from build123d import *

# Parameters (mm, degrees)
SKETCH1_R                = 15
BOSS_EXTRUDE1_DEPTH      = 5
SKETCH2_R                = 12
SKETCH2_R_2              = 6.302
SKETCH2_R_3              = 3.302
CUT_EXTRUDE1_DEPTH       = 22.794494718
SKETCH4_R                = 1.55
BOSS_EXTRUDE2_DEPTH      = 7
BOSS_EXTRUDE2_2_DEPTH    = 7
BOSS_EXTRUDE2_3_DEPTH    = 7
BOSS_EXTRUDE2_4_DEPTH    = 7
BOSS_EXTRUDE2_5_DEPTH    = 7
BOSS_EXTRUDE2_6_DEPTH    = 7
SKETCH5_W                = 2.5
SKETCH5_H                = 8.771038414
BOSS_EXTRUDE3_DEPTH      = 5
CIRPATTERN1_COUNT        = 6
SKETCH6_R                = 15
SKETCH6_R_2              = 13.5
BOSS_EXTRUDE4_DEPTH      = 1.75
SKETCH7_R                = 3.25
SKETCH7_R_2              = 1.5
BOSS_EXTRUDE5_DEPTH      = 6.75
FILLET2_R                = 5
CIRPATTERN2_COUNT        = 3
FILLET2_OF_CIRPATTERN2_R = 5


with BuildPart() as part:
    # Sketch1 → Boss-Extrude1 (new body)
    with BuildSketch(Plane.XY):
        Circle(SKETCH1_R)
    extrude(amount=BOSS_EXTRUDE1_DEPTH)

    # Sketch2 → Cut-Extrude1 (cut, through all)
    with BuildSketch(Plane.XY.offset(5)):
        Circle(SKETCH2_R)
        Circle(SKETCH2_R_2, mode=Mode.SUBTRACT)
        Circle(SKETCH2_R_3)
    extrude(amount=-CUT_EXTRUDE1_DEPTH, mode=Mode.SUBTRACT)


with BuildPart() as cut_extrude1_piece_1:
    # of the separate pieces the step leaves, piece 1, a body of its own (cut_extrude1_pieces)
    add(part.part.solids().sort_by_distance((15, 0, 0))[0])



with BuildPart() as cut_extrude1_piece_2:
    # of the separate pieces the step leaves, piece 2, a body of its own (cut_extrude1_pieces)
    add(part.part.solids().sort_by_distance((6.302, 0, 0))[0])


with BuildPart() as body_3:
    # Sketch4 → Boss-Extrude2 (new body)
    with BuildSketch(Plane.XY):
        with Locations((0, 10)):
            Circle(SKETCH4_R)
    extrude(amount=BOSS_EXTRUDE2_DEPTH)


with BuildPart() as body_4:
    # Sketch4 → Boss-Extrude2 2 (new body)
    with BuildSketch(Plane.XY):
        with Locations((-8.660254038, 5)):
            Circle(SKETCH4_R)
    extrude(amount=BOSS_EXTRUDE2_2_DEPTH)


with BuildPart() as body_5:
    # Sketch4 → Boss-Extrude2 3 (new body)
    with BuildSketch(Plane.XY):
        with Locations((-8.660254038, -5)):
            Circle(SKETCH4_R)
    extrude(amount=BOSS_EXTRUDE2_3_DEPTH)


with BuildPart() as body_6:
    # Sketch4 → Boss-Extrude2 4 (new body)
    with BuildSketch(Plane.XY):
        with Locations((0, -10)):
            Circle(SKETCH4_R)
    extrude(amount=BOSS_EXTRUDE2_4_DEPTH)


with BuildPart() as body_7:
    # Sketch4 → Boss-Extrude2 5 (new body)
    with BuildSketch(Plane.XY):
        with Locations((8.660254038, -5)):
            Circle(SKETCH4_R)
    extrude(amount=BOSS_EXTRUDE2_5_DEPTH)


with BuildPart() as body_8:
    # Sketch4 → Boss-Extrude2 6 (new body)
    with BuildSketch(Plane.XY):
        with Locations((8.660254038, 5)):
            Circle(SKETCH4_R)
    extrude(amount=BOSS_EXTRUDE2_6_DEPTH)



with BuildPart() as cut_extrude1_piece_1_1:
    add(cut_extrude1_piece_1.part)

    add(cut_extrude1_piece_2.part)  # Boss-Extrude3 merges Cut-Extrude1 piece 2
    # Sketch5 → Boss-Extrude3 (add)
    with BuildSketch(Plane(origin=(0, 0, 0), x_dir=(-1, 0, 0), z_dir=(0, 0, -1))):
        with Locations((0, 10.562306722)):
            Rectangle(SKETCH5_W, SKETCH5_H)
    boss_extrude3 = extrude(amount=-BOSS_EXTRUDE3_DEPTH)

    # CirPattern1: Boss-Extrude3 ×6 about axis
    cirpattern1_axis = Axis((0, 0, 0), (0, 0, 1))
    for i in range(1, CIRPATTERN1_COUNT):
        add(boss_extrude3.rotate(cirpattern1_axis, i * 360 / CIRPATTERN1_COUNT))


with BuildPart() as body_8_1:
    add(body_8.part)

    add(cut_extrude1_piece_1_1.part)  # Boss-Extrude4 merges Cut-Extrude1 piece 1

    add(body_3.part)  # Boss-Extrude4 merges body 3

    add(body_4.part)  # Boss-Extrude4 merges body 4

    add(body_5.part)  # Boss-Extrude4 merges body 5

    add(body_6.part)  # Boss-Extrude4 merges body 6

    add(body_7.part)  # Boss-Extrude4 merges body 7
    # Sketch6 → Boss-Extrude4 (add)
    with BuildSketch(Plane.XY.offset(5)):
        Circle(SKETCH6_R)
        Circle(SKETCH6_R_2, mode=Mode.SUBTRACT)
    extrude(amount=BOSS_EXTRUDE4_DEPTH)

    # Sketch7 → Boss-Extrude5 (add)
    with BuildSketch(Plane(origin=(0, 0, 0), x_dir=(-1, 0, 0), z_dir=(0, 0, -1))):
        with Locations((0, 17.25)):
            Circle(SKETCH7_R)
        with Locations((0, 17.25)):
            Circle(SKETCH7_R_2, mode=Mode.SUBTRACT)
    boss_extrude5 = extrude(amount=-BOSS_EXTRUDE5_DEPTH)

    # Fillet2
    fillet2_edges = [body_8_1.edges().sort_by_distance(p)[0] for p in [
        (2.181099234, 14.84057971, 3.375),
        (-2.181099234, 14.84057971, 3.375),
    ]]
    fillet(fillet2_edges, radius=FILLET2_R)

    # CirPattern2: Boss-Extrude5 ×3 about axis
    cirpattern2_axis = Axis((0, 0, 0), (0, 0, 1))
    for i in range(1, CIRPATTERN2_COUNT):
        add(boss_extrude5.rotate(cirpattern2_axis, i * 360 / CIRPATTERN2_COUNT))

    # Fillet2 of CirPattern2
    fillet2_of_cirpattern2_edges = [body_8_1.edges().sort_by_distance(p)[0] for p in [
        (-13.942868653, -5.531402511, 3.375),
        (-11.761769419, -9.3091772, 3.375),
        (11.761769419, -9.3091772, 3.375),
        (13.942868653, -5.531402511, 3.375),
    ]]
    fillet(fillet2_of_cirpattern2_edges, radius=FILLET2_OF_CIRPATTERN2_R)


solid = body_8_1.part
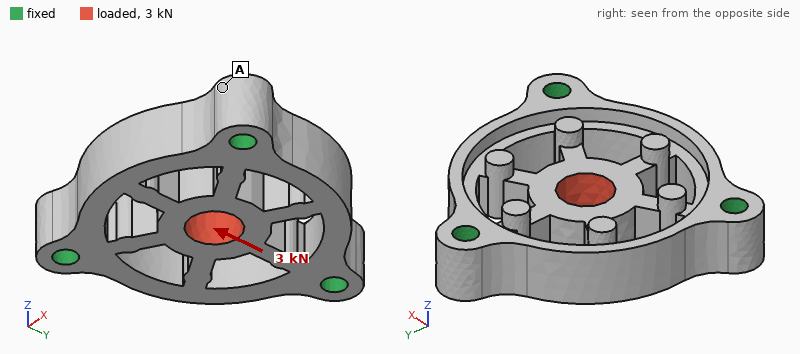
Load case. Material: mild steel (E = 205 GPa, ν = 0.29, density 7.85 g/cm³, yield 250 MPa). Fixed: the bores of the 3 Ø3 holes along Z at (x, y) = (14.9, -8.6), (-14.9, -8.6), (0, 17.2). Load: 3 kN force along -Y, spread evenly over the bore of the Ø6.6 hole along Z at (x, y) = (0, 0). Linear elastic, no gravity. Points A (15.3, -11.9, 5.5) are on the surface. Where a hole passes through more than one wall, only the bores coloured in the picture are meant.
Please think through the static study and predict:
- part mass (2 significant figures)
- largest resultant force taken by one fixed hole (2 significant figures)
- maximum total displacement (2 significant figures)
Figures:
24 g
1.1 kN
7.8 µm
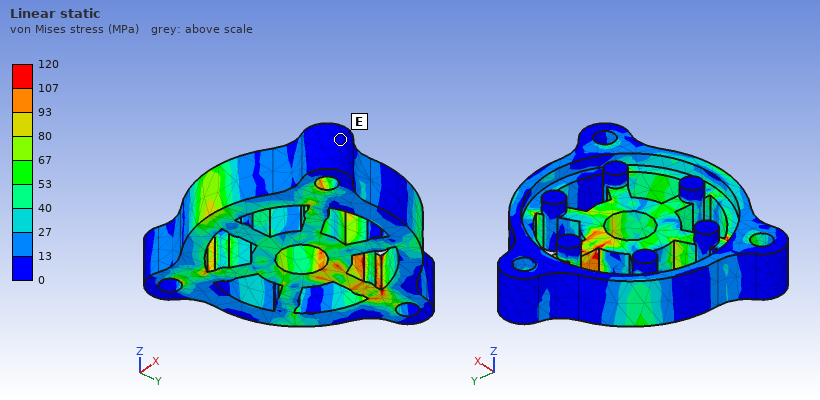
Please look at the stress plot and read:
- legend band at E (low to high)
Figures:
0 to 13 MPa
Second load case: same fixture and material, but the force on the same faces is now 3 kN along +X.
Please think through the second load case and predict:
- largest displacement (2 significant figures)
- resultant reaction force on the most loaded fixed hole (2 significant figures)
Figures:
7.5 µm
1.0 kN
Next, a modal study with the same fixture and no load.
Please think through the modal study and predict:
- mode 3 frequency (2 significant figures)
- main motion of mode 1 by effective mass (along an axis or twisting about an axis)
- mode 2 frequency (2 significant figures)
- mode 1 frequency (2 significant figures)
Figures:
28 kHz
along Z
28 kHz
25 kHz
